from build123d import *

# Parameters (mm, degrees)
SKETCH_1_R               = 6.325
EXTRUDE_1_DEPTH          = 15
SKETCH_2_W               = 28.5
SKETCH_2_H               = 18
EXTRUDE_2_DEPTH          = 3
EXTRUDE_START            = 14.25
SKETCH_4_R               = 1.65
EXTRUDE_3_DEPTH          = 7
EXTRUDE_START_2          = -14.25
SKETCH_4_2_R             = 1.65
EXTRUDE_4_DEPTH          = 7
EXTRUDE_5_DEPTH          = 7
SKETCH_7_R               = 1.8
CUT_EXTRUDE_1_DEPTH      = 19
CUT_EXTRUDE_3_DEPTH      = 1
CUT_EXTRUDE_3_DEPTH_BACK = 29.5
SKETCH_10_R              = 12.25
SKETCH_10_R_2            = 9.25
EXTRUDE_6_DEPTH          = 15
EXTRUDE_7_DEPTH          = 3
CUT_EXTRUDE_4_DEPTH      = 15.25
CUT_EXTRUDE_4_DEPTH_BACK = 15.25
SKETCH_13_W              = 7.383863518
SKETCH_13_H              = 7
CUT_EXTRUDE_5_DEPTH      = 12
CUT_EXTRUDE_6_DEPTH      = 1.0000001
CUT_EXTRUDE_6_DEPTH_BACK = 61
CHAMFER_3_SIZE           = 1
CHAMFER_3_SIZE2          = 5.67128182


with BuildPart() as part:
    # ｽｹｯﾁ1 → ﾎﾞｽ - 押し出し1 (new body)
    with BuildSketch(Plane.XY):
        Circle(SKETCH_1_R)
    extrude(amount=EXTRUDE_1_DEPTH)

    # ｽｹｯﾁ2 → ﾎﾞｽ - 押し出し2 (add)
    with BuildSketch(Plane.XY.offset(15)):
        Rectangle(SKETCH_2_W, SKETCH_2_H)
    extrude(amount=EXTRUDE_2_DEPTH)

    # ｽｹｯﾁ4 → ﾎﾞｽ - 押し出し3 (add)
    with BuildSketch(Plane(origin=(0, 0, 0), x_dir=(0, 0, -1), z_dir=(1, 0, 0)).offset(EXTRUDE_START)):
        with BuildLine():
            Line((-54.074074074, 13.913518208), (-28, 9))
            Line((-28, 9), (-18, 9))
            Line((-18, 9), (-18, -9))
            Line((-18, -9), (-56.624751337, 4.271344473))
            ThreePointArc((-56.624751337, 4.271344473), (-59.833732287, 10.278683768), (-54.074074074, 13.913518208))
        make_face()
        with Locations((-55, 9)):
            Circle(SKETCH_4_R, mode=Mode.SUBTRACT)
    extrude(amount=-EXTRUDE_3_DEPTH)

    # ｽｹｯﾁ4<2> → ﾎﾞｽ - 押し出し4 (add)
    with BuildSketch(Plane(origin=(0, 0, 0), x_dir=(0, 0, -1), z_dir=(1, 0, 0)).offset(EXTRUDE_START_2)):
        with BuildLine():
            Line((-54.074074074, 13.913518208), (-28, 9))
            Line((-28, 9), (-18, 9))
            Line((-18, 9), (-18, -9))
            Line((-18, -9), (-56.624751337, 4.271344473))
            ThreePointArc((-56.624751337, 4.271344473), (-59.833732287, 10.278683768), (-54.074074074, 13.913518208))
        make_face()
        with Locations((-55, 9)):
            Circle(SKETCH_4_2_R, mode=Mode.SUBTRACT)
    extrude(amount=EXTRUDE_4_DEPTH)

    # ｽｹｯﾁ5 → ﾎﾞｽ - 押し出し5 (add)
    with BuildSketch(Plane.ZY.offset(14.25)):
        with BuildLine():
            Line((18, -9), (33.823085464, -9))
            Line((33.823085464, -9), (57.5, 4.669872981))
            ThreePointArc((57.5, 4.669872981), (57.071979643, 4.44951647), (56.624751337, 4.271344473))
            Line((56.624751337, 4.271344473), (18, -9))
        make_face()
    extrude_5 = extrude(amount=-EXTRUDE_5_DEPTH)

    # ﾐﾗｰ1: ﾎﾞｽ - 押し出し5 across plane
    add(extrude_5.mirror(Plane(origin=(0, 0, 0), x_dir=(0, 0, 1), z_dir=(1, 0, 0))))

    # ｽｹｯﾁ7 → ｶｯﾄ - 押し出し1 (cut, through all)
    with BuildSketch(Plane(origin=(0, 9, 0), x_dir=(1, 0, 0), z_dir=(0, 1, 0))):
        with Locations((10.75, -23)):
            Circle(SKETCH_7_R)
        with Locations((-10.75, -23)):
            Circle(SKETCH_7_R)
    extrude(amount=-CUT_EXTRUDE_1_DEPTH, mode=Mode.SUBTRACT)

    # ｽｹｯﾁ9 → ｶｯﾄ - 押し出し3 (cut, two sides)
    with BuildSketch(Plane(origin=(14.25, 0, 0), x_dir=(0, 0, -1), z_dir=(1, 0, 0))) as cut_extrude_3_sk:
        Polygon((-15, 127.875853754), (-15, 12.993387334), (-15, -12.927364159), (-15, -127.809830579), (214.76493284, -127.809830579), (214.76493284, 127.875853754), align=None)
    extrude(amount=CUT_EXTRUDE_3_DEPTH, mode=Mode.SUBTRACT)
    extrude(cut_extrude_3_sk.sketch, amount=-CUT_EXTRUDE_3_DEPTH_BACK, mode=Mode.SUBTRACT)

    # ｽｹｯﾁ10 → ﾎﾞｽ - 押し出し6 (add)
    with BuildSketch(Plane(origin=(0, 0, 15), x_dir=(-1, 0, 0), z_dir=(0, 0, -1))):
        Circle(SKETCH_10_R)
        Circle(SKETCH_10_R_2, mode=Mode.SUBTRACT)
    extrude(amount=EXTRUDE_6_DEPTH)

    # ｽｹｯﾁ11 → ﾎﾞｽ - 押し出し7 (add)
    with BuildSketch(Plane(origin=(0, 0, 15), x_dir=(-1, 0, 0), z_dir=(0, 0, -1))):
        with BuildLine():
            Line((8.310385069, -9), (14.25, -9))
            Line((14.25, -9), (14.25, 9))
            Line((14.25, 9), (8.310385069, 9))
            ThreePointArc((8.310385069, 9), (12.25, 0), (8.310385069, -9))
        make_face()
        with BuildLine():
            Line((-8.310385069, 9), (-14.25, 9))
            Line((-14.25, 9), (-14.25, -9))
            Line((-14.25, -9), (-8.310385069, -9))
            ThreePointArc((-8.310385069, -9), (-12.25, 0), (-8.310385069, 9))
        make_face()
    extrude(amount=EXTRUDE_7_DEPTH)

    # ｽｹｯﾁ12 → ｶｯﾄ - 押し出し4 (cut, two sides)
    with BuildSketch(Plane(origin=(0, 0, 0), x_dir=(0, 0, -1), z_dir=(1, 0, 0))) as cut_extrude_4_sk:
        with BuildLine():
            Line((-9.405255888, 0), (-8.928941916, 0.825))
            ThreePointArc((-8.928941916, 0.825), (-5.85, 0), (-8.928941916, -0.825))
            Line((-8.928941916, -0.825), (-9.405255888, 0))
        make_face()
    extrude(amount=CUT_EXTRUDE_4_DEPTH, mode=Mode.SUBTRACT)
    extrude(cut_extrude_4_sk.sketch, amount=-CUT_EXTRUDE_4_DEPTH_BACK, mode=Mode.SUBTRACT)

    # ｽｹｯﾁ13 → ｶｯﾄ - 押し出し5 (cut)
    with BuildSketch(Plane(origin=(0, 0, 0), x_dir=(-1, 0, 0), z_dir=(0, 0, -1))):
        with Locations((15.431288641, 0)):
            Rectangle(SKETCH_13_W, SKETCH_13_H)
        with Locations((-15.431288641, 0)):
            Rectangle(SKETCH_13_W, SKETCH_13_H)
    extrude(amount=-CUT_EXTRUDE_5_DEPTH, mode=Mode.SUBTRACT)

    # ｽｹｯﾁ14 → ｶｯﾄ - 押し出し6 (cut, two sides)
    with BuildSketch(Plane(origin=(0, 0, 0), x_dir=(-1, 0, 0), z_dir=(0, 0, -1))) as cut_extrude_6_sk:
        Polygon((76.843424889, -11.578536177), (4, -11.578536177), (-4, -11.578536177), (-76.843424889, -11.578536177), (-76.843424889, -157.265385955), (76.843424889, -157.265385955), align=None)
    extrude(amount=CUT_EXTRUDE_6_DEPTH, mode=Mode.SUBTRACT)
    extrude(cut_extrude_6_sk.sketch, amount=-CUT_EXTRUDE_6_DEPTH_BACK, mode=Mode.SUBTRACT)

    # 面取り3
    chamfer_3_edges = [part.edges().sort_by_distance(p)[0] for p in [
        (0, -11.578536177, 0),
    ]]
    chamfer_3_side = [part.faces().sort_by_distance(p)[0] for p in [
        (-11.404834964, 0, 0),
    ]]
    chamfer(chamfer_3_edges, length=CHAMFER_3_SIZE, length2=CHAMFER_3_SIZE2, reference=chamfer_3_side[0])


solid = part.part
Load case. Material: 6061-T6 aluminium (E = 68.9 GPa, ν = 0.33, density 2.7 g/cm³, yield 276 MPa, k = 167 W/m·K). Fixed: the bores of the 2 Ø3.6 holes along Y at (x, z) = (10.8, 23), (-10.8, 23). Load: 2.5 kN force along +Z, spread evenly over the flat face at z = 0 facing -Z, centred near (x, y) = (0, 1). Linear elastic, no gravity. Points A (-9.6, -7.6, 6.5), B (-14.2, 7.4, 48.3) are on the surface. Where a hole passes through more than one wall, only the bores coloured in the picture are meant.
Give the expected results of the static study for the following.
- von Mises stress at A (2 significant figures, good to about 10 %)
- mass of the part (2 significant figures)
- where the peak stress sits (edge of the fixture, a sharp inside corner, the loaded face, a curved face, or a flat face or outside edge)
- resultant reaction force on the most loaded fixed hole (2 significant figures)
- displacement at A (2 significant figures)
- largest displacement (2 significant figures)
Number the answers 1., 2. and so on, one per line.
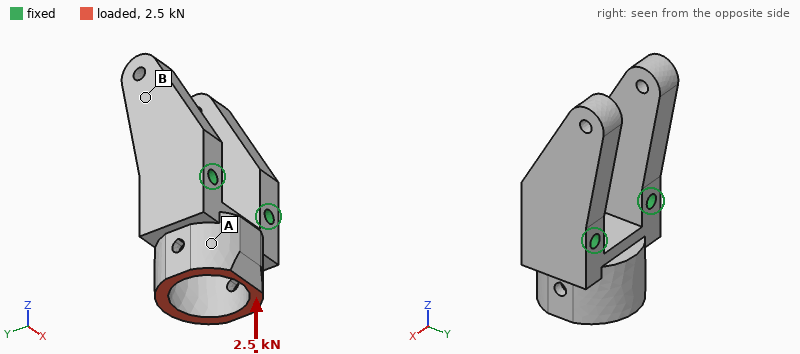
1. 17 MPa
2. 36 g
3. a curved face
4. 1.3 kN
5. 3.4 µm
6. 13 µm
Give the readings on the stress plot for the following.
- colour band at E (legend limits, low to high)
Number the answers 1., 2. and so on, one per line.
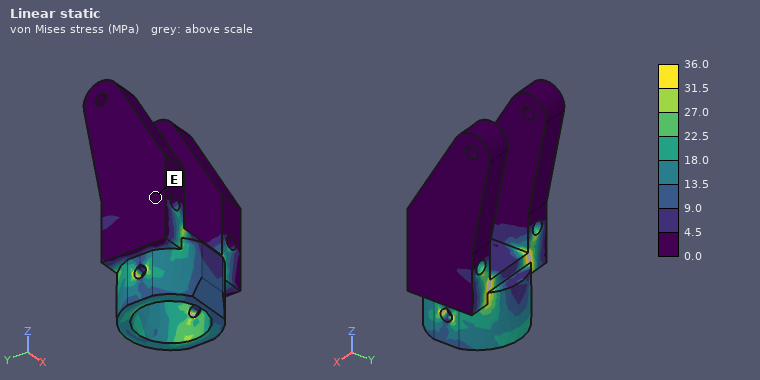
1. 0.0 to 4.5 MPa
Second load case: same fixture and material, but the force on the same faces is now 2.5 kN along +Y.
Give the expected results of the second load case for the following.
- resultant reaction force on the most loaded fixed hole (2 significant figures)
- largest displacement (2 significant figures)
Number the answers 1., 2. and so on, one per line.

1. 1.3 kN
2. 69 µm
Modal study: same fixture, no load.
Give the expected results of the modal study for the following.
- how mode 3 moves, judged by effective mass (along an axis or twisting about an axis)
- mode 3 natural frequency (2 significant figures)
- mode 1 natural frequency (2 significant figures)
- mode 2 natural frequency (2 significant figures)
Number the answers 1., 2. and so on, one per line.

1. along Y
2. 12 kHz
3. 5100 Hz
4. 5100 Hz
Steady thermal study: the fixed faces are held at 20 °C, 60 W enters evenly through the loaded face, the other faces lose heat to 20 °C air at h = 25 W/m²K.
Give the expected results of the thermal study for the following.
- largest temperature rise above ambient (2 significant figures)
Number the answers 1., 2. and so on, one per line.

1. 42 K
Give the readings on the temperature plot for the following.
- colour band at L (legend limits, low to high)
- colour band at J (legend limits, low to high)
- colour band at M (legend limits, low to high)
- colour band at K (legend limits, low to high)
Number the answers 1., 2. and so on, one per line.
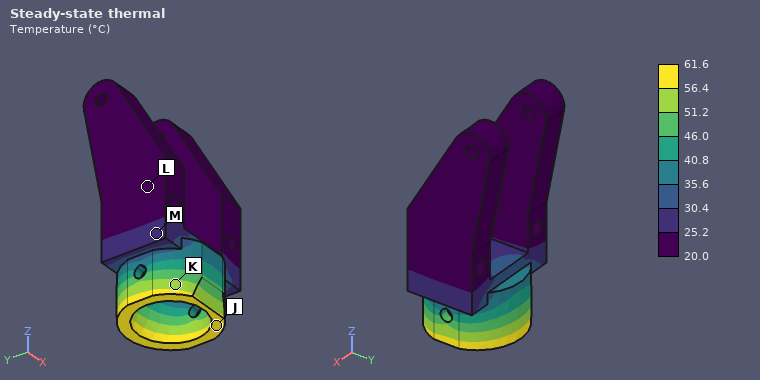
1. 20.0 to 25.2 °C
2. 56.4 to 61.6 °C
3. 25.2 to 30.4 °C
4. 51.2 to 56.4 °C
